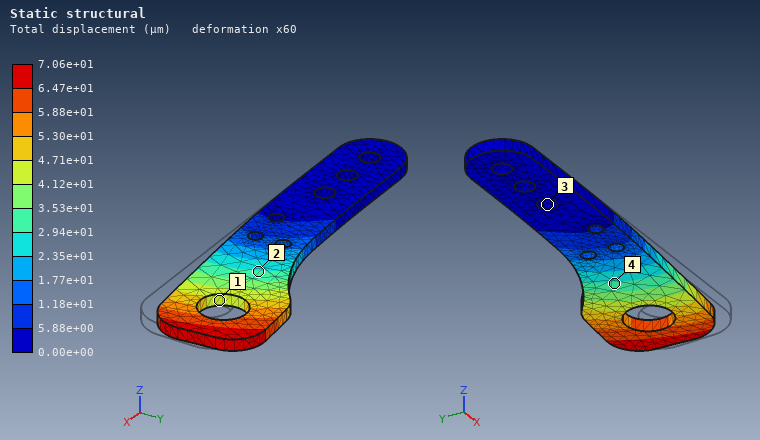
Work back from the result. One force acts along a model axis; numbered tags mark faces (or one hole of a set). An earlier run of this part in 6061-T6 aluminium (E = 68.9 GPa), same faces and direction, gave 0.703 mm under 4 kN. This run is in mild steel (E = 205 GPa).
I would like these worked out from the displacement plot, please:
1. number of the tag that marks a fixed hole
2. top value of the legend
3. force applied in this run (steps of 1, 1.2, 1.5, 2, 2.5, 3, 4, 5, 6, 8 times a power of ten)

3
7.06e+01 µm
1.2 kN
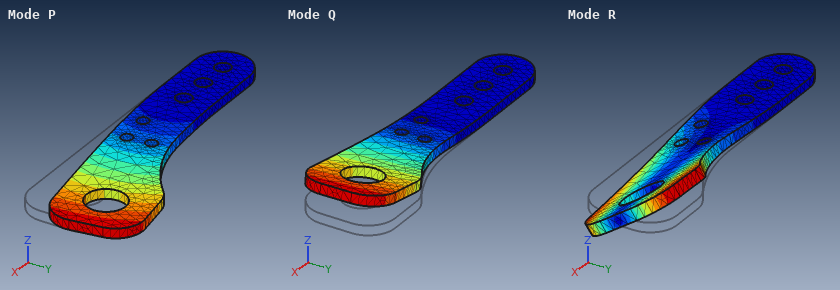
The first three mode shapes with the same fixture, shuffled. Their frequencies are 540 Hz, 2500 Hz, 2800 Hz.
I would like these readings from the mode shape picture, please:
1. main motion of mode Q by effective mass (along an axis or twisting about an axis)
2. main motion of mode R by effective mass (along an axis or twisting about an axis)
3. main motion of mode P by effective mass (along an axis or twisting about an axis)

along Z
twisting about X
along Y
